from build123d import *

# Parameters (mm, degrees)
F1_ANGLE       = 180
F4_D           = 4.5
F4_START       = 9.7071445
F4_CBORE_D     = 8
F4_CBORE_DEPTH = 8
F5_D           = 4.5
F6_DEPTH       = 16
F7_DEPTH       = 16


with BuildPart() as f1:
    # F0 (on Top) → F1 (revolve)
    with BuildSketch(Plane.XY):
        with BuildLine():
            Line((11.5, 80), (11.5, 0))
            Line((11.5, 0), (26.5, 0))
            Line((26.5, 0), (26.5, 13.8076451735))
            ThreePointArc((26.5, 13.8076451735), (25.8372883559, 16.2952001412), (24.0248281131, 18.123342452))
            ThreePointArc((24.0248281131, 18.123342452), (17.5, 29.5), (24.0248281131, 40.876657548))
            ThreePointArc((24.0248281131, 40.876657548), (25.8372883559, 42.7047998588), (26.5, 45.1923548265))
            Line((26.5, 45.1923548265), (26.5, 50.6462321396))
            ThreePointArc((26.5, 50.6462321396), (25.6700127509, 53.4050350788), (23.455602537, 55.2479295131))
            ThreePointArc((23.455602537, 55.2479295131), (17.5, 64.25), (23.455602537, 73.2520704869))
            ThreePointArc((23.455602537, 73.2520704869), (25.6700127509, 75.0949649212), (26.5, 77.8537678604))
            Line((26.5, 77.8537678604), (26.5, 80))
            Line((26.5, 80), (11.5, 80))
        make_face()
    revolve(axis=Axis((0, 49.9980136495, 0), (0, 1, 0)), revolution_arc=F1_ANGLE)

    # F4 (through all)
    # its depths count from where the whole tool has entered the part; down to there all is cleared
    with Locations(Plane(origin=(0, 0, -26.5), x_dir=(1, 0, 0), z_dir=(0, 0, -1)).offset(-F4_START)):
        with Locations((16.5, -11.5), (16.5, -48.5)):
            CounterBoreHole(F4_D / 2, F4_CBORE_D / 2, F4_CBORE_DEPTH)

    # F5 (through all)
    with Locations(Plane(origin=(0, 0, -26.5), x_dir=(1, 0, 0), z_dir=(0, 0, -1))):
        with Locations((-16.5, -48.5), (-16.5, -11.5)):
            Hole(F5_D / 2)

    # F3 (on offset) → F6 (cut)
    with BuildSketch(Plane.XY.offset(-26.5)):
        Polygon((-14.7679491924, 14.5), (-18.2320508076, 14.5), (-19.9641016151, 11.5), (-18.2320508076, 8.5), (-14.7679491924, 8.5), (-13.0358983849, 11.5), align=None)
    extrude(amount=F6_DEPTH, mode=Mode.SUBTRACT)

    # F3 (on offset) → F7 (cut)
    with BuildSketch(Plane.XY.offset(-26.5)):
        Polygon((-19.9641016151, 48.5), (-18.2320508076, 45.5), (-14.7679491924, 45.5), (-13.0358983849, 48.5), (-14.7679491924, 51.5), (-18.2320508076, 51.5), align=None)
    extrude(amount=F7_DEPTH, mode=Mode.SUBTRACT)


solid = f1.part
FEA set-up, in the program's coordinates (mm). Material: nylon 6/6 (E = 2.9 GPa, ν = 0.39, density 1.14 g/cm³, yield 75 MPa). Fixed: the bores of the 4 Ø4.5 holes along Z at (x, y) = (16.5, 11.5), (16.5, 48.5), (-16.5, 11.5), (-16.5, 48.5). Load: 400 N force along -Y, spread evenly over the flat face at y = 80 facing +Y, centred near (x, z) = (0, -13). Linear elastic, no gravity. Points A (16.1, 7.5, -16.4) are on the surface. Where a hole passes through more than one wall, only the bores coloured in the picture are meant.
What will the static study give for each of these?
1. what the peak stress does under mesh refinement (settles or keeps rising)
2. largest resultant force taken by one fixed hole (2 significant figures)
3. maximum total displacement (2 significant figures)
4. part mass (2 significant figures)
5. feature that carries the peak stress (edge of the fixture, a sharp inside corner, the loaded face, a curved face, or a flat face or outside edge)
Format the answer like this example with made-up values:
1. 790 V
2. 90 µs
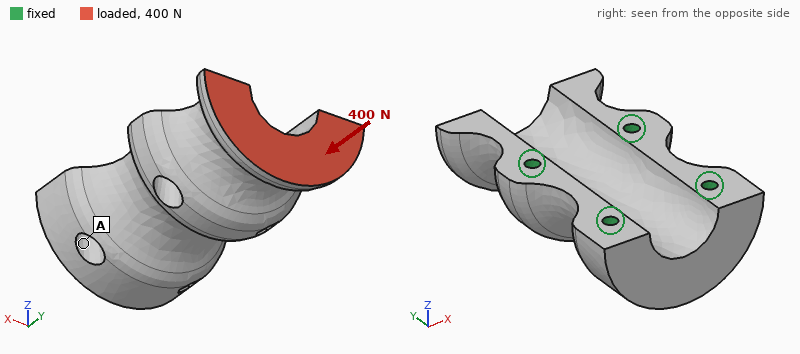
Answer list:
1. keeps rising
2. 150 N
3. 74 µm
4. 54 g
5. edge of the fixture
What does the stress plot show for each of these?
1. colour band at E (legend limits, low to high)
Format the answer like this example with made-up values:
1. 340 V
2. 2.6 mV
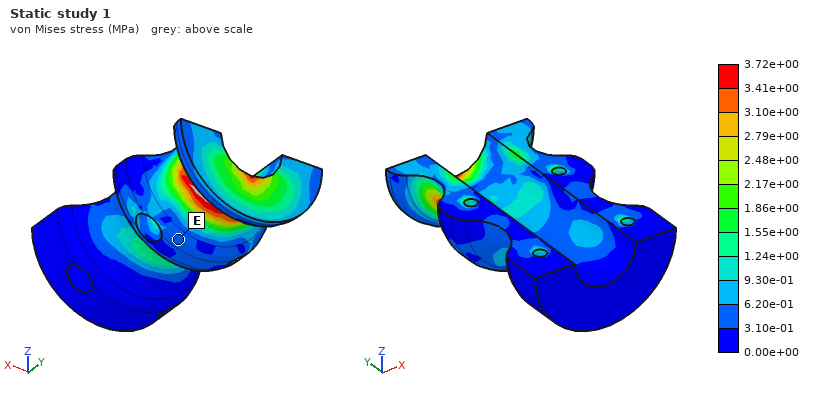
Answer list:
1. 3.10e-01 to 6.20e-01 MPa
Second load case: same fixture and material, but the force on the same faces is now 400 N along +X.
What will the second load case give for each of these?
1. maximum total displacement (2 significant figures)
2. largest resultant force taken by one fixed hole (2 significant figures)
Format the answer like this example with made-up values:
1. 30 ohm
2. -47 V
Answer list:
1. 0.22 mm
2. 410 N
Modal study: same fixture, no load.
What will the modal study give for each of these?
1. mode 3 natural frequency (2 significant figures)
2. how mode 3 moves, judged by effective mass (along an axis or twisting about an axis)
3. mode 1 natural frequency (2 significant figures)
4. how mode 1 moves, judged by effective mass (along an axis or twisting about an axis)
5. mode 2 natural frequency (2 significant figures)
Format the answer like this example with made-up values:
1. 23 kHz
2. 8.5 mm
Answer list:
1. 4200 Hz
2. along X
3. 2300 Hz
4. along Z
5. 2400 Hz
